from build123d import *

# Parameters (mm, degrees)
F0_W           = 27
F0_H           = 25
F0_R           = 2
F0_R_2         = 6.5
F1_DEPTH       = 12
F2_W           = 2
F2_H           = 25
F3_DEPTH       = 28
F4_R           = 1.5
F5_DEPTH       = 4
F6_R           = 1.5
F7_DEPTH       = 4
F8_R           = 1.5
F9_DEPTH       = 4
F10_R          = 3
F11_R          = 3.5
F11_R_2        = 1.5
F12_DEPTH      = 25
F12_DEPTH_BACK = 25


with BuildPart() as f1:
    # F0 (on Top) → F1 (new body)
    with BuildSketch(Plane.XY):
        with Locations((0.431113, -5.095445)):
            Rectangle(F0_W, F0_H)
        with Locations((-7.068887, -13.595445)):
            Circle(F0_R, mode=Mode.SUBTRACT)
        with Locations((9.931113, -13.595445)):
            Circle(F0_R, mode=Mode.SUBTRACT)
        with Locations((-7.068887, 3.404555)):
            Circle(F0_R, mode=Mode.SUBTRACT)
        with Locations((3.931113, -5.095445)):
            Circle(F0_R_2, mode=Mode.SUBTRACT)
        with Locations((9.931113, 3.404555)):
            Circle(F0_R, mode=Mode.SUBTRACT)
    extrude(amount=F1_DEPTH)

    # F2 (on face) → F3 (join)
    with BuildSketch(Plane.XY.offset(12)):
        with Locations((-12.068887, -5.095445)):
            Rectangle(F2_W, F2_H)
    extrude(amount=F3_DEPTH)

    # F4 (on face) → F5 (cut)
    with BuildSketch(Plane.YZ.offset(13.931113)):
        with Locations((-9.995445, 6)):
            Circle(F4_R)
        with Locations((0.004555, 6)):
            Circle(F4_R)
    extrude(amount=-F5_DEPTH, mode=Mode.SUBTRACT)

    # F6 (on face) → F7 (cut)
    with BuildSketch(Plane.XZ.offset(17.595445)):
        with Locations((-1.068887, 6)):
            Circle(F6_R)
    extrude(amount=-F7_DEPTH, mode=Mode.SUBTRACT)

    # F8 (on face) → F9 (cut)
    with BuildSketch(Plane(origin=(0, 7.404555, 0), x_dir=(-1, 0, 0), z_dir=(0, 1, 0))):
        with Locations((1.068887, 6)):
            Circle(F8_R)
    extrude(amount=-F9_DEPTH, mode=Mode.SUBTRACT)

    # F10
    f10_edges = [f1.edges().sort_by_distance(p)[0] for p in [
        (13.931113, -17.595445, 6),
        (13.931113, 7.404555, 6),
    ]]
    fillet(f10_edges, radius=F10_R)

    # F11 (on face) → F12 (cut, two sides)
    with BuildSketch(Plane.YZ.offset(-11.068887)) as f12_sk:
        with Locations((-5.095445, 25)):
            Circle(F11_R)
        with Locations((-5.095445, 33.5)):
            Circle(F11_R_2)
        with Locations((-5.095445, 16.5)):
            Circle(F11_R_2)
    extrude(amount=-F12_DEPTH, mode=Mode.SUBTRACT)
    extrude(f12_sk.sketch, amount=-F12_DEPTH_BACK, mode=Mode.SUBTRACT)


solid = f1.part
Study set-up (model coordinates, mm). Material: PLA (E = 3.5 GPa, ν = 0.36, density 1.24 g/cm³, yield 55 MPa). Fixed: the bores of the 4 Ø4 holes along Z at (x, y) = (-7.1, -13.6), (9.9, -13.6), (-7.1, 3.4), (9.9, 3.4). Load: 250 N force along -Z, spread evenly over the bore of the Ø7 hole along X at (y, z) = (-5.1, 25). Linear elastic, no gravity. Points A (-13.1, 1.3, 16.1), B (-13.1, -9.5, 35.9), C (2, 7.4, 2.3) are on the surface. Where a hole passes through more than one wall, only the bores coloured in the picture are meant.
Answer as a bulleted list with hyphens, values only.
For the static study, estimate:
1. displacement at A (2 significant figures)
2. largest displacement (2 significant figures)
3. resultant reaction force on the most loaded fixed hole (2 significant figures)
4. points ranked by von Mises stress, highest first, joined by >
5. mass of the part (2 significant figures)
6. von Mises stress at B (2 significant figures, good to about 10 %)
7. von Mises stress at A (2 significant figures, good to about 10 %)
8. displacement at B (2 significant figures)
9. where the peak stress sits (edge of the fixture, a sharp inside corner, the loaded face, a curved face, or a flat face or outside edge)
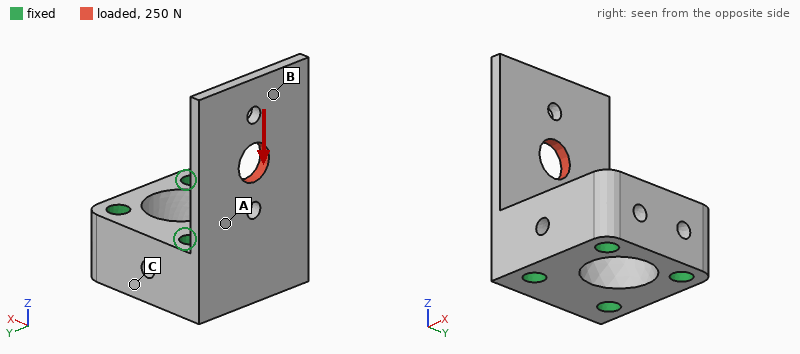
- 23 µm
- 78 µm
- 130 N
- A > B > C
- 8.7 g
- 2.5 MPa
- 5.6 MPa
- 69 µm
- a curved face
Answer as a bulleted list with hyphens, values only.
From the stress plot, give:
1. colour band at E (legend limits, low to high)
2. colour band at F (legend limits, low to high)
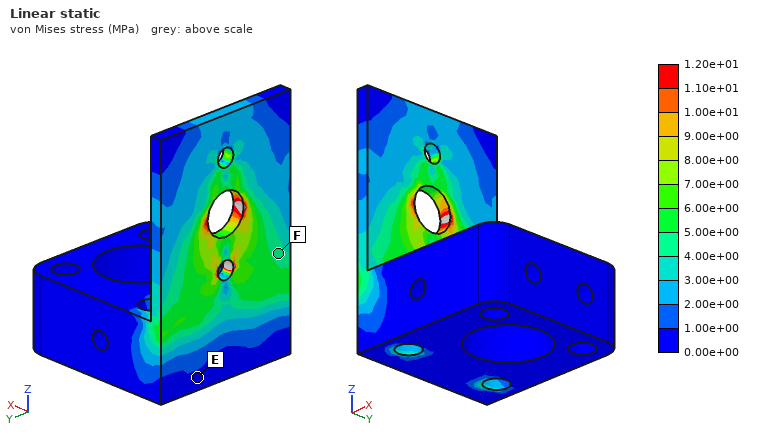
- 0.00e+00 to 1.00e+00 MPa
- 4.00e+00 to 5.00e+00 MPa
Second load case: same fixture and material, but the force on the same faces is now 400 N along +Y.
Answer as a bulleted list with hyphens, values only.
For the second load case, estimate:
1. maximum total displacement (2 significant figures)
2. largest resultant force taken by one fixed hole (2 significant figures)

- 0.37 mm
- 390 N
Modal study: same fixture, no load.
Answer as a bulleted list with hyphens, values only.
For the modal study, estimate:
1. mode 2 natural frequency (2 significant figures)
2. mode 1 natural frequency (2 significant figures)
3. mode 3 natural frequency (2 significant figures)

- 1600 Hz
- 640 Hz
- 3900 Hz
